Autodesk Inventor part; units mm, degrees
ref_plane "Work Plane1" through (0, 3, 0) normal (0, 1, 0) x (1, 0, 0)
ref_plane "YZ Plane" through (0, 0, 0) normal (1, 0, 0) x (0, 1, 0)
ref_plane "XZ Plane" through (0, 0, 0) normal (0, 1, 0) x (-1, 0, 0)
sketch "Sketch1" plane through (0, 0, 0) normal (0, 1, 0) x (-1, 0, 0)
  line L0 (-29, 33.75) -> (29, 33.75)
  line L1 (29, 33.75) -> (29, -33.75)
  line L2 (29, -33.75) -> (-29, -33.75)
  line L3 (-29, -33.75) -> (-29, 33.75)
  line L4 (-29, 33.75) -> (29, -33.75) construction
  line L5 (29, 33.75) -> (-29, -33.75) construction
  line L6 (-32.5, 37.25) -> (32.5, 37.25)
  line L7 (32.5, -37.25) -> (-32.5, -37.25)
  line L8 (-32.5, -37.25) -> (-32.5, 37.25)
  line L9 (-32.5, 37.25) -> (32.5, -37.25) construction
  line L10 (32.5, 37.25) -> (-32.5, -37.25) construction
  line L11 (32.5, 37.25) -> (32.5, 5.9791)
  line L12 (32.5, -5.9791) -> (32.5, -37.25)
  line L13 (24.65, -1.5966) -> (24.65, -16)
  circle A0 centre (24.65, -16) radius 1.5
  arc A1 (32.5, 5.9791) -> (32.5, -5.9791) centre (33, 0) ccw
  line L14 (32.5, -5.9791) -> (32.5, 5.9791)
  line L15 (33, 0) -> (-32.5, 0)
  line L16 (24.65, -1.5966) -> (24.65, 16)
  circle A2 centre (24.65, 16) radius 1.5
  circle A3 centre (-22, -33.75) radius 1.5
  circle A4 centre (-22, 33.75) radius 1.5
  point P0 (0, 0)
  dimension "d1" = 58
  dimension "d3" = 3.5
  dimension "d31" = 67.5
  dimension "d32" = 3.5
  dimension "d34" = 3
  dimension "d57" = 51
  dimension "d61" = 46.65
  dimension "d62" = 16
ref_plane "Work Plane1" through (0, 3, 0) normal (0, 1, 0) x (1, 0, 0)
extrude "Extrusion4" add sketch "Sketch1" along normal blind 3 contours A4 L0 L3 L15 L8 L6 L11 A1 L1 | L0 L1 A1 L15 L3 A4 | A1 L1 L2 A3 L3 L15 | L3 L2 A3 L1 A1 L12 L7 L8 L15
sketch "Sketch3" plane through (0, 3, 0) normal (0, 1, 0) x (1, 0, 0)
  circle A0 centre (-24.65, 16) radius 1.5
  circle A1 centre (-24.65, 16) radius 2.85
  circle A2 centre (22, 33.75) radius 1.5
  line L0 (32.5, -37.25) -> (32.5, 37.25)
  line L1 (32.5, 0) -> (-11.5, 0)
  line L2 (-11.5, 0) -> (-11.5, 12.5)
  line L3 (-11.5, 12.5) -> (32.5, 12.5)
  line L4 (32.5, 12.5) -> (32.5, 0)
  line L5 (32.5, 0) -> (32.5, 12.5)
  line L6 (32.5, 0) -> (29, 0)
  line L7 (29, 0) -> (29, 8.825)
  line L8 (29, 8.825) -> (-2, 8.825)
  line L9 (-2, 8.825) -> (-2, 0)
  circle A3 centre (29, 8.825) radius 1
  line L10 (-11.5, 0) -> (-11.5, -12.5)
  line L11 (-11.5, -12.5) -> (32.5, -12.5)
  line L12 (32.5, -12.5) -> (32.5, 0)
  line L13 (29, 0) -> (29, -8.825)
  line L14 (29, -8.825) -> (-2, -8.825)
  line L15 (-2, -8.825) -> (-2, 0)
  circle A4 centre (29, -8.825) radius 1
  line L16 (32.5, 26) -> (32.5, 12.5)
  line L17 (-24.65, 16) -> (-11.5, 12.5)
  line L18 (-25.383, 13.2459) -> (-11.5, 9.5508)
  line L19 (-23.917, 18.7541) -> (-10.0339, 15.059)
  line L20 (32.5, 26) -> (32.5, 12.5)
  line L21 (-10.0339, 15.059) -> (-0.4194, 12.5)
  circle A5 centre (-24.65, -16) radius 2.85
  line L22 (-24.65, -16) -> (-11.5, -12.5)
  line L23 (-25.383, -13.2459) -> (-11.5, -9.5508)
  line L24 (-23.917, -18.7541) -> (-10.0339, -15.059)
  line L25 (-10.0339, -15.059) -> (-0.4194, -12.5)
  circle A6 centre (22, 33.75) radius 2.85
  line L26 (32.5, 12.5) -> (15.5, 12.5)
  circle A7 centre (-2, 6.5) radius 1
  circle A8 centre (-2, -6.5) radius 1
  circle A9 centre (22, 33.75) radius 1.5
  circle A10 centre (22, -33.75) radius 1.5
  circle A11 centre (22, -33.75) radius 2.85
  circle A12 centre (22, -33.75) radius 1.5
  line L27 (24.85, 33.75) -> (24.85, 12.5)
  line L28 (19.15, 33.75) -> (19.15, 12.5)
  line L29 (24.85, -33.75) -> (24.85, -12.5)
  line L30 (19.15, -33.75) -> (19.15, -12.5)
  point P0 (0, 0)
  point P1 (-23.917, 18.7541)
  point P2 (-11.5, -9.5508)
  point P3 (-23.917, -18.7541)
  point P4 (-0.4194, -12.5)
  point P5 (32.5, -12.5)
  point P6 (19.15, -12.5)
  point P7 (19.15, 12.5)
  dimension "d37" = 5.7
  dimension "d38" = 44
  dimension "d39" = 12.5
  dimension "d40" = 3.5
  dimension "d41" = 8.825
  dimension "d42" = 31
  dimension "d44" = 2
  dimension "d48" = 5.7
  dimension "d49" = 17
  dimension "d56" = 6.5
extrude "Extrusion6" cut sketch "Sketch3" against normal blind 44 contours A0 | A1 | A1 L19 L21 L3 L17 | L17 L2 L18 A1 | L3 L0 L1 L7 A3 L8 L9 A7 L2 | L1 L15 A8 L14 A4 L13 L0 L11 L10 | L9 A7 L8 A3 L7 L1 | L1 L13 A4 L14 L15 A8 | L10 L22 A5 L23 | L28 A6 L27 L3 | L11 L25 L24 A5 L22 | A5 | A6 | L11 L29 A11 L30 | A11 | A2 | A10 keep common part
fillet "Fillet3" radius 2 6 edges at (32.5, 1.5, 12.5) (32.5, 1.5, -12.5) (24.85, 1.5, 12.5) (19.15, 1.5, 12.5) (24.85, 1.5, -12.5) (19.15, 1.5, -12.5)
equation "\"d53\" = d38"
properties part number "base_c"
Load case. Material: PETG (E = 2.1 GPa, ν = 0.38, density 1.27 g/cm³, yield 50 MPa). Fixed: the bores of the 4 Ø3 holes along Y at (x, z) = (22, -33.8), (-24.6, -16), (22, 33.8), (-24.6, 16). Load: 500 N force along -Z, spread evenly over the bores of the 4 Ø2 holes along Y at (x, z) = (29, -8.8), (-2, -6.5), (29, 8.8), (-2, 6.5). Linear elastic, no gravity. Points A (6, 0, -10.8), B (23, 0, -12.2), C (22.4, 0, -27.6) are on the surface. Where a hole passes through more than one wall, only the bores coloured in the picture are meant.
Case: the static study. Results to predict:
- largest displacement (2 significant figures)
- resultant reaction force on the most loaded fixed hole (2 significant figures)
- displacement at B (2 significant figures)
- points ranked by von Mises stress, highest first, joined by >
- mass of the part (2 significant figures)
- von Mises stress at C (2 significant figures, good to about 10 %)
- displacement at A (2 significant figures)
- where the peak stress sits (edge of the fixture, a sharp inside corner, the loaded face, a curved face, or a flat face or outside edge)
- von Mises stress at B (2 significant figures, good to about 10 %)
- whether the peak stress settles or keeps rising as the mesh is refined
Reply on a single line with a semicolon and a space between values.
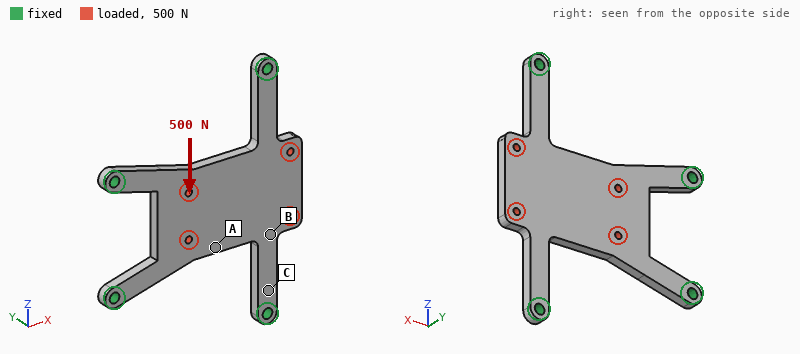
0.30 mm; 180 N; 0.11 mm; C > B > A; 5.9 g; 11 MPa; 0.22 mm; edge of the fixture; 5.9 MPa; keeps rising
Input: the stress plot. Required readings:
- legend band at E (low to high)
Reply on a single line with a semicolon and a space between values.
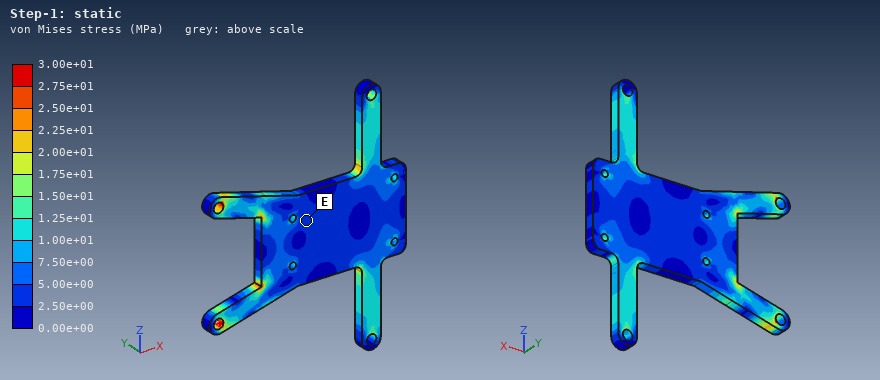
2.50e+00 to 5.00e+00 MPa
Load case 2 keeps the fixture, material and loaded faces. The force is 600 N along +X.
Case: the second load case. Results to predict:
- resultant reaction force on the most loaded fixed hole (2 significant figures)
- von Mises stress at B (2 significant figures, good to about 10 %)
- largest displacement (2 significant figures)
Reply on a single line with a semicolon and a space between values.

290 N; 3.3 MPa; 0.26 mm
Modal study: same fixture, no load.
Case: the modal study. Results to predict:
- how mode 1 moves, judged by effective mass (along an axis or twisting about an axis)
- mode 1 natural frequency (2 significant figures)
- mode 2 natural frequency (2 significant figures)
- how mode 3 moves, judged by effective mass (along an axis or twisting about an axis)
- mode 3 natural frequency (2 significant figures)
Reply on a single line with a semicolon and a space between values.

along Y; 610 Hz; 1200 Hz; twisting about X; 1800 Hz
